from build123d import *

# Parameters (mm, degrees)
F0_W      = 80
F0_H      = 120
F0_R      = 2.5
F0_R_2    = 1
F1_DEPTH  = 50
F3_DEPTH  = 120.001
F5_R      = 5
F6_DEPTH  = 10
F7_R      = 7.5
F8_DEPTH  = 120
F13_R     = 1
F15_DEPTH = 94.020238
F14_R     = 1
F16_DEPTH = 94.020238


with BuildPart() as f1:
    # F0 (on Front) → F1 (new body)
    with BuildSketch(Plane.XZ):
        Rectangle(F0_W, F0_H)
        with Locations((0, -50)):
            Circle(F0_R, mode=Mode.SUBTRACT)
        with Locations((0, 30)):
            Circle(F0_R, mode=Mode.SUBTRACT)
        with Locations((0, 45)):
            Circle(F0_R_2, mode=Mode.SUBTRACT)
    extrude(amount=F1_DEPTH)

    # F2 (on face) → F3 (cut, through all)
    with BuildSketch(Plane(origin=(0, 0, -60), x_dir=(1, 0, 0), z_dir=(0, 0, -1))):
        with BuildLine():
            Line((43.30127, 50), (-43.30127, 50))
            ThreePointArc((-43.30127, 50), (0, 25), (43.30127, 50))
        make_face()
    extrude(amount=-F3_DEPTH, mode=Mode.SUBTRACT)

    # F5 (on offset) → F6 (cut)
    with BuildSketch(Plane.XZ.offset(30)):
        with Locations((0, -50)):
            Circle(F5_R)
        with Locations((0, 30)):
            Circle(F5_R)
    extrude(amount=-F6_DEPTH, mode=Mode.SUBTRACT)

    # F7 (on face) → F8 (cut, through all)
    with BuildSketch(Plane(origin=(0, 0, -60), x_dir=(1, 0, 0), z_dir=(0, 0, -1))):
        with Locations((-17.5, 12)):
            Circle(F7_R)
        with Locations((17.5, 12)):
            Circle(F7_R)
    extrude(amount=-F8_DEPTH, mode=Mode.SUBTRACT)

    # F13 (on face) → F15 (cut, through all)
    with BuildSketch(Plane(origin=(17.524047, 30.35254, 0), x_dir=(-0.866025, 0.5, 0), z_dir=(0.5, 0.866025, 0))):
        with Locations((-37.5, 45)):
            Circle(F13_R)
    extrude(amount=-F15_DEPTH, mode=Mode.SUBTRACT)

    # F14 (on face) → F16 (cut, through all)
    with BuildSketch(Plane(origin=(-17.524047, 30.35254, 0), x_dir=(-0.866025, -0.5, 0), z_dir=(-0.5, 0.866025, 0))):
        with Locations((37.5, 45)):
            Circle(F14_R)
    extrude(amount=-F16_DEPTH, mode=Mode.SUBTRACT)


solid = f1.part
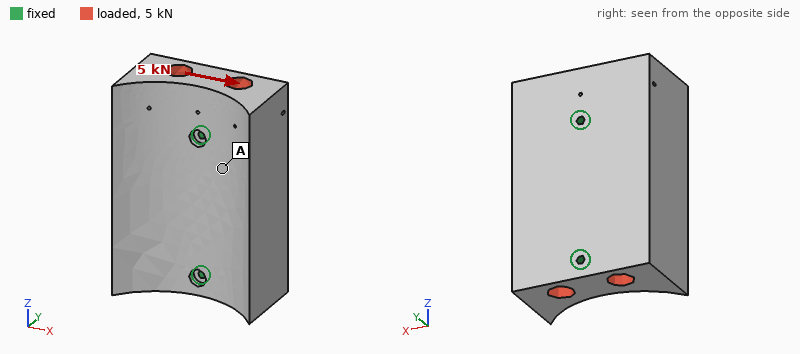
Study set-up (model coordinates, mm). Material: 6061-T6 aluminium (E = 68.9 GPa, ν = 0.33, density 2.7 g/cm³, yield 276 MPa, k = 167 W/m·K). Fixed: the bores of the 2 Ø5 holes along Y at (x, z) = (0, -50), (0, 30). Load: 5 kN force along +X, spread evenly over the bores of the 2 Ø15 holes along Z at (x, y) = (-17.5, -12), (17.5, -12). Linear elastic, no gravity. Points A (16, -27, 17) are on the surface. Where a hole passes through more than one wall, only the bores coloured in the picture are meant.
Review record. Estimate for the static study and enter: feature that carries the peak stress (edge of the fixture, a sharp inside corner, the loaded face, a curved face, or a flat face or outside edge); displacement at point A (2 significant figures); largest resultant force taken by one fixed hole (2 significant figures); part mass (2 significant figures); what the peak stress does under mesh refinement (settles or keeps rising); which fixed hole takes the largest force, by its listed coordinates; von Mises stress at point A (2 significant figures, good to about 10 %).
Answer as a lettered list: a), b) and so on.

a) edge of the fixture
b) 2.4 µm
c) 3.1 kN
d) 680 g
e) keeps rising
f) (0, 30)
g) 1.8 MPa
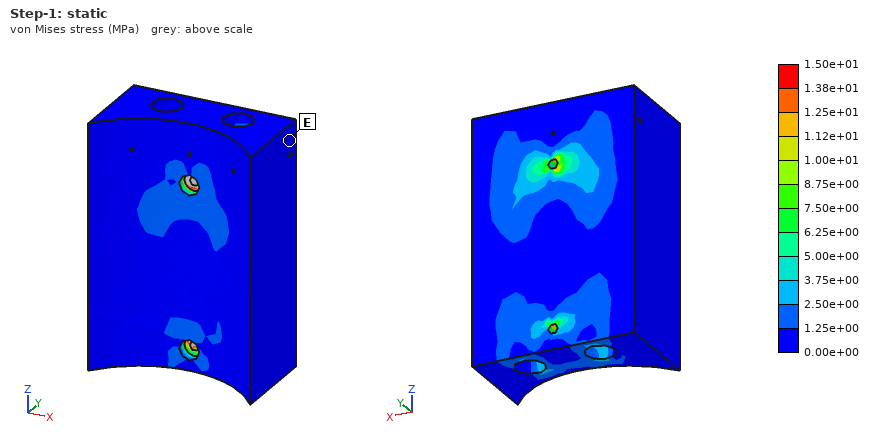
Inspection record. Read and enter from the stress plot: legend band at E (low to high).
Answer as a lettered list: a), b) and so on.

a) 0.00e+00 to 1.25e+00 MPa
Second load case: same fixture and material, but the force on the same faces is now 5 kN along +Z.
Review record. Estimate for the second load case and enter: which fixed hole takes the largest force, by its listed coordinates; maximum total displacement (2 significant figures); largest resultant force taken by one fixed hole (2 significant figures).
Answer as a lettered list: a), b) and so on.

a) (0, 30)
b) 1.9 µm
c) 2.9 kN
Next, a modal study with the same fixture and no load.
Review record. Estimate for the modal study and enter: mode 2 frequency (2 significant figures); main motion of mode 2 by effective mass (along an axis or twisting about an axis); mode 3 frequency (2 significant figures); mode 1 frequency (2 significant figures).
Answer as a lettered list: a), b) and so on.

a) 5600 Hz
b) along Y
c) 6700 Hz
d) 3100 Hz
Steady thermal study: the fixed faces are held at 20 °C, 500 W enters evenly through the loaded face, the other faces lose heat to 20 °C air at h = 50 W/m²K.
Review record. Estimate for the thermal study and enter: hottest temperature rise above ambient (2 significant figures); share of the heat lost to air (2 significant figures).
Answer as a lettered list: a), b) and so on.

a) 32 K
b) 9.7 %
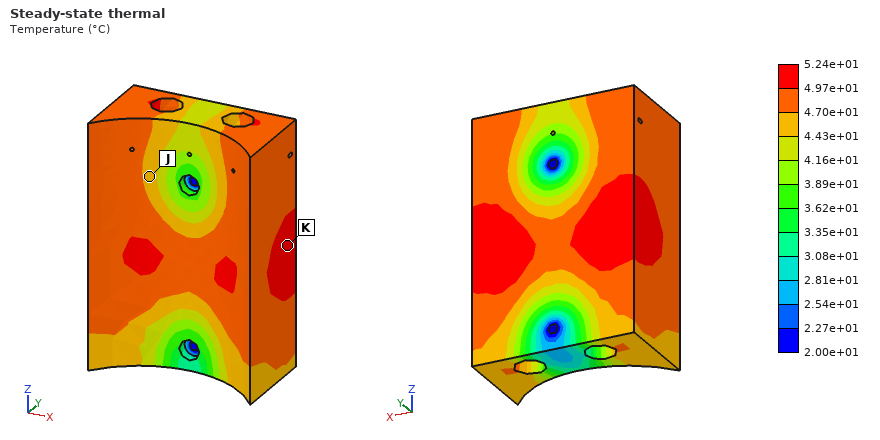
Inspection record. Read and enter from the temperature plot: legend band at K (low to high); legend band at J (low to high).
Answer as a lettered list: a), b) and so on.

a) 4.97e+01 to 5.24e+01 °C
b) 4.43e+01 to 4.70e+01 °C
